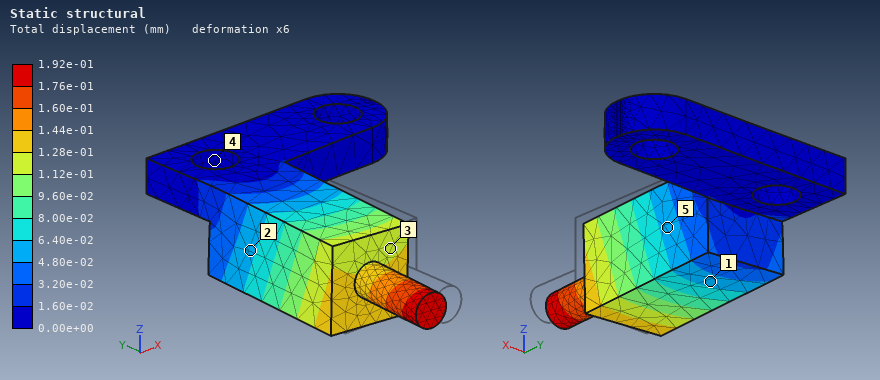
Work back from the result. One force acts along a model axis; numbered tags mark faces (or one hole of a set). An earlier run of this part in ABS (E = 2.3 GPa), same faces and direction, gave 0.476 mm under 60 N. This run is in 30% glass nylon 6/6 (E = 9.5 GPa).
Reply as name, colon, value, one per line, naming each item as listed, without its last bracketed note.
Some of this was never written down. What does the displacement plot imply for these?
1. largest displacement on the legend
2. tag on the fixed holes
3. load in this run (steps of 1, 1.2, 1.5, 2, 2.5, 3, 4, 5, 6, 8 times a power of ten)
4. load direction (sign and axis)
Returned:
largest displacement on the legend: 1.92e-01 mm
tag on the fixed holes: 4
load in this run: 100 N
load direction: -X
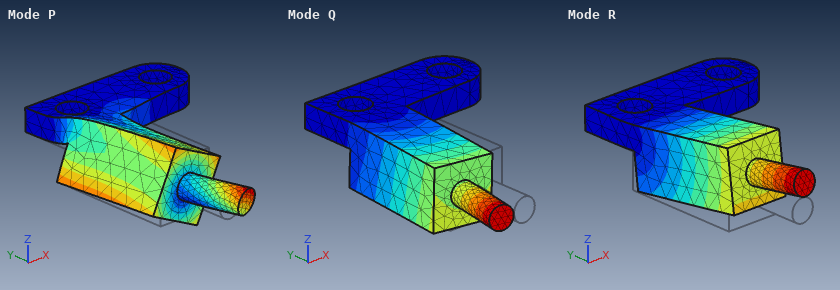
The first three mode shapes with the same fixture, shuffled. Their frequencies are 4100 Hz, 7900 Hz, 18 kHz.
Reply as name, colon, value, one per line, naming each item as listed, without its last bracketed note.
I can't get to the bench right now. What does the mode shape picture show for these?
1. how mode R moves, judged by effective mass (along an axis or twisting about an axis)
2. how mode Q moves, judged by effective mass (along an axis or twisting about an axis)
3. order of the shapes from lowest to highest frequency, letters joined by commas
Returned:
how mode R moves, judged by effective mass: along Z
how mode Q moves, judged by effective mass: along X
order of the shapes from lowest to highest frequency, letters joined by commas: R, Q, P
